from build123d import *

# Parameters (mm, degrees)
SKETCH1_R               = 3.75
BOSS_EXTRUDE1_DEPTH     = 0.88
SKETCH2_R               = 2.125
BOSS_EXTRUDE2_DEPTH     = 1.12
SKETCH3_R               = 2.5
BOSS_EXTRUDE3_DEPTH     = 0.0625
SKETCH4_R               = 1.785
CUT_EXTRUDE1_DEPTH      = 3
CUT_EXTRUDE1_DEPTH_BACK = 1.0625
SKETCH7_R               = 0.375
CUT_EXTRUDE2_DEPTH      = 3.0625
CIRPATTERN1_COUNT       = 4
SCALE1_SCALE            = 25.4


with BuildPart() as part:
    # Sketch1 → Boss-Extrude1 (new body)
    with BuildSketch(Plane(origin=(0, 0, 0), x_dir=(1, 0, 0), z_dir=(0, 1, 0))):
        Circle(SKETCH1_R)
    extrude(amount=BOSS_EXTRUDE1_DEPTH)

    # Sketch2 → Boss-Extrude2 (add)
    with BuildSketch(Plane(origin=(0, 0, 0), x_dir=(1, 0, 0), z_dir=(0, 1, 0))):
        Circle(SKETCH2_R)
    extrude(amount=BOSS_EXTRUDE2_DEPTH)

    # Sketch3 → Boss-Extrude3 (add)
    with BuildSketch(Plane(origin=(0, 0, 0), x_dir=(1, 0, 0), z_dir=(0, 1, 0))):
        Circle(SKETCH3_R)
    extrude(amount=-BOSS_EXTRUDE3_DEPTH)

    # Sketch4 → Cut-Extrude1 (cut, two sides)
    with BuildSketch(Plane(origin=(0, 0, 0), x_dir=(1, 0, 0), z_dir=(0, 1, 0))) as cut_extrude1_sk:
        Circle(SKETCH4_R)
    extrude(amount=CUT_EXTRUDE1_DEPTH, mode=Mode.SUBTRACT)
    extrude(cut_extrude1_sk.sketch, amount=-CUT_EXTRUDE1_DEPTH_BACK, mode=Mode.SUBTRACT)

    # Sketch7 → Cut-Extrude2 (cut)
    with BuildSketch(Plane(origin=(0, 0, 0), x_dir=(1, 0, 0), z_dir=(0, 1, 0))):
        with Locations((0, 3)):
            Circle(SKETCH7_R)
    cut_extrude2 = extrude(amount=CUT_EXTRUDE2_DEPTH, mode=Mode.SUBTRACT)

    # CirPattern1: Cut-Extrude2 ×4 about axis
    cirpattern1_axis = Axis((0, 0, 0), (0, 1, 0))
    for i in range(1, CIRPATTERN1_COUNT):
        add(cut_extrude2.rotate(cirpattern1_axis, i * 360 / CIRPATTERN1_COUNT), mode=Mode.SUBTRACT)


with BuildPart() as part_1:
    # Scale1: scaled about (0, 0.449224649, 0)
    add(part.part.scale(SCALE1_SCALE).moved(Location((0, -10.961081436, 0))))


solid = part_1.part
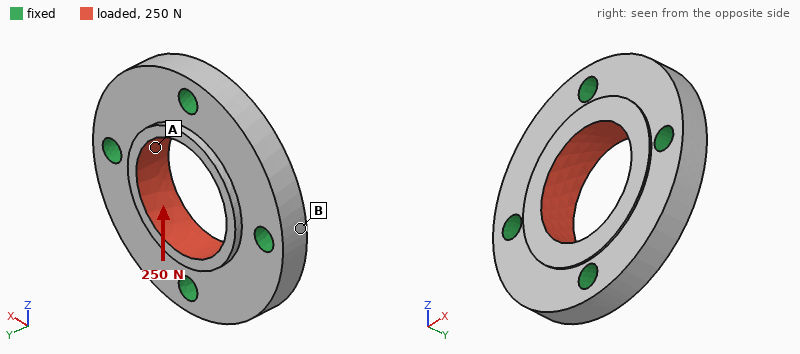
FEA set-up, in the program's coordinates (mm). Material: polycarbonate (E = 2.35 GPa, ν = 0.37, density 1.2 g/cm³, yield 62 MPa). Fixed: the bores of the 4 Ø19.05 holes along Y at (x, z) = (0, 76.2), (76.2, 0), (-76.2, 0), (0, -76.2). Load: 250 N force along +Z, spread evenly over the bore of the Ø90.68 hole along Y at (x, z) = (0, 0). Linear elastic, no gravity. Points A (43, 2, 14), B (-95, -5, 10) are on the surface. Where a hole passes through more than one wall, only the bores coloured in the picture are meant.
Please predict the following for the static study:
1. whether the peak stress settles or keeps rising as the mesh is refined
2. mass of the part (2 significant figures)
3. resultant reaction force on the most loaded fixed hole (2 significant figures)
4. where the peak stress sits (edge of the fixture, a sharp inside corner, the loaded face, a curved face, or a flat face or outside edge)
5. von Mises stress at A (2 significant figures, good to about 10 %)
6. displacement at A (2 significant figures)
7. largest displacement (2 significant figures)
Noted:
keeps rising
590 g
64 N
edge of the fixture
0.053 MPa
1.4 µm
1.9 µm
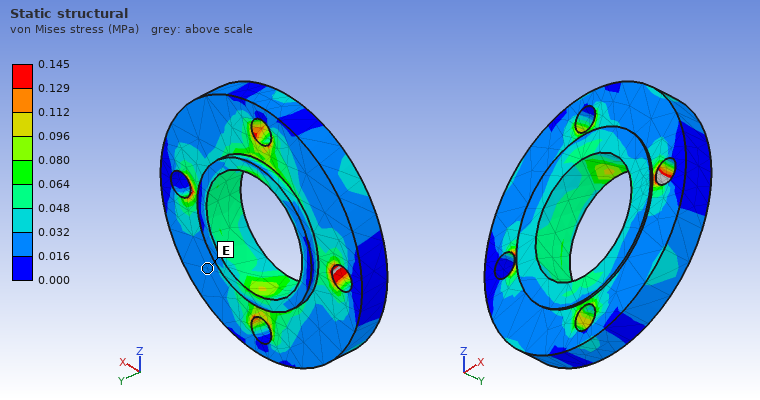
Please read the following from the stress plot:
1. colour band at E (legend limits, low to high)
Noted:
0.016 to 0.032 MPa
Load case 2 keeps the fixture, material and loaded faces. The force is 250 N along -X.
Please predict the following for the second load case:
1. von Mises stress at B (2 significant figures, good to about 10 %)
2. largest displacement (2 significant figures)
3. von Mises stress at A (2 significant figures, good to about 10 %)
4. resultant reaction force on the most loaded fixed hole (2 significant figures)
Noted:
0.030 MPa
1.9 µm
0.050 MPa
64 N
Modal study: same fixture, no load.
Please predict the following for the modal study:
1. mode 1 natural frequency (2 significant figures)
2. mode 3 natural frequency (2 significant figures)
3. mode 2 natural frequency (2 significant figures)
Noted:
2000 Hz
2000 Hz
2000 Hz
